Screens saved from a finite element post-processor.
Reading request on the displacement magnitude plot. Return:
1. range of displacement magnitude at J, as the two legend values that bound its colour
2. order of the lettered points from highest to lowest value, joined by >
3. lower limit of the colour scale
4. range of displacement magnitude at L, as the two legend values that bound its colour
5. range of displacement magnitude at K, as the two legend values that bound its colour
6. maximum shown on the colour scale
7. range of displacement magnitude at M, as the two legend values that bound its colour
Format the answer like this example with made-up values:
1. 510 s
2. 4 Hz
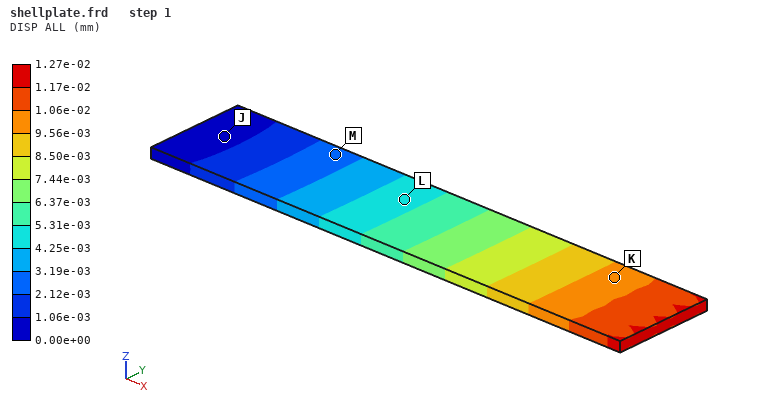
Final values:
1. 0.00e+00 to 1.06e-03 mm
2. K > L > M > J
3. 0.00e+00 mm
4. 4.25e-03 to 5.31e-03 mm
5. 9.56e-03 to 1.06e-02 mm
6. 1.27e-02 mm
7. 2.12e-03 to 3.19e-03 mm
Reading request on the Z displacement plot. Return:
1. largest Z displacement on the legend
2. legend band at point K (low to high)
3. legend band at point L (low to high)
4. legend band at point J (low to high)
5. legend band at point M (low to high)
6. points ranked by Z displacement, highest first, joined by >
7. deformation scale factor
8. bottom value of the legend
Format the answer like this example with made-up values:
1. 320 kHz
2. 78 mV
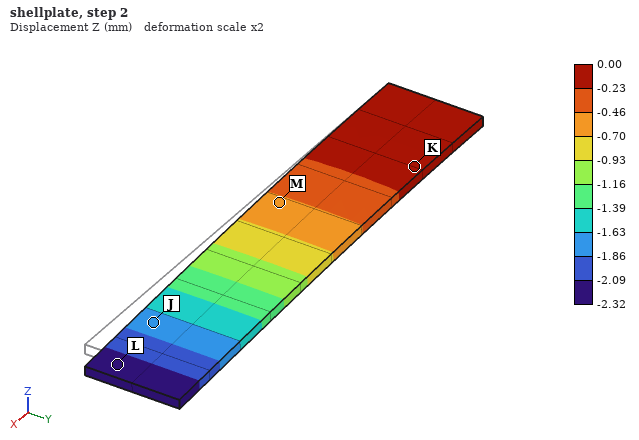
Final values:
1. 0.00 mm
2. -0.23 to 0.00 mm
3. -2.32 to -2.09 mm
4. -1.86 to -1.63 mm
5. -0.70 to -0.46 mm
6. K > M > J > L
7. 2
8. -2.32 mm
